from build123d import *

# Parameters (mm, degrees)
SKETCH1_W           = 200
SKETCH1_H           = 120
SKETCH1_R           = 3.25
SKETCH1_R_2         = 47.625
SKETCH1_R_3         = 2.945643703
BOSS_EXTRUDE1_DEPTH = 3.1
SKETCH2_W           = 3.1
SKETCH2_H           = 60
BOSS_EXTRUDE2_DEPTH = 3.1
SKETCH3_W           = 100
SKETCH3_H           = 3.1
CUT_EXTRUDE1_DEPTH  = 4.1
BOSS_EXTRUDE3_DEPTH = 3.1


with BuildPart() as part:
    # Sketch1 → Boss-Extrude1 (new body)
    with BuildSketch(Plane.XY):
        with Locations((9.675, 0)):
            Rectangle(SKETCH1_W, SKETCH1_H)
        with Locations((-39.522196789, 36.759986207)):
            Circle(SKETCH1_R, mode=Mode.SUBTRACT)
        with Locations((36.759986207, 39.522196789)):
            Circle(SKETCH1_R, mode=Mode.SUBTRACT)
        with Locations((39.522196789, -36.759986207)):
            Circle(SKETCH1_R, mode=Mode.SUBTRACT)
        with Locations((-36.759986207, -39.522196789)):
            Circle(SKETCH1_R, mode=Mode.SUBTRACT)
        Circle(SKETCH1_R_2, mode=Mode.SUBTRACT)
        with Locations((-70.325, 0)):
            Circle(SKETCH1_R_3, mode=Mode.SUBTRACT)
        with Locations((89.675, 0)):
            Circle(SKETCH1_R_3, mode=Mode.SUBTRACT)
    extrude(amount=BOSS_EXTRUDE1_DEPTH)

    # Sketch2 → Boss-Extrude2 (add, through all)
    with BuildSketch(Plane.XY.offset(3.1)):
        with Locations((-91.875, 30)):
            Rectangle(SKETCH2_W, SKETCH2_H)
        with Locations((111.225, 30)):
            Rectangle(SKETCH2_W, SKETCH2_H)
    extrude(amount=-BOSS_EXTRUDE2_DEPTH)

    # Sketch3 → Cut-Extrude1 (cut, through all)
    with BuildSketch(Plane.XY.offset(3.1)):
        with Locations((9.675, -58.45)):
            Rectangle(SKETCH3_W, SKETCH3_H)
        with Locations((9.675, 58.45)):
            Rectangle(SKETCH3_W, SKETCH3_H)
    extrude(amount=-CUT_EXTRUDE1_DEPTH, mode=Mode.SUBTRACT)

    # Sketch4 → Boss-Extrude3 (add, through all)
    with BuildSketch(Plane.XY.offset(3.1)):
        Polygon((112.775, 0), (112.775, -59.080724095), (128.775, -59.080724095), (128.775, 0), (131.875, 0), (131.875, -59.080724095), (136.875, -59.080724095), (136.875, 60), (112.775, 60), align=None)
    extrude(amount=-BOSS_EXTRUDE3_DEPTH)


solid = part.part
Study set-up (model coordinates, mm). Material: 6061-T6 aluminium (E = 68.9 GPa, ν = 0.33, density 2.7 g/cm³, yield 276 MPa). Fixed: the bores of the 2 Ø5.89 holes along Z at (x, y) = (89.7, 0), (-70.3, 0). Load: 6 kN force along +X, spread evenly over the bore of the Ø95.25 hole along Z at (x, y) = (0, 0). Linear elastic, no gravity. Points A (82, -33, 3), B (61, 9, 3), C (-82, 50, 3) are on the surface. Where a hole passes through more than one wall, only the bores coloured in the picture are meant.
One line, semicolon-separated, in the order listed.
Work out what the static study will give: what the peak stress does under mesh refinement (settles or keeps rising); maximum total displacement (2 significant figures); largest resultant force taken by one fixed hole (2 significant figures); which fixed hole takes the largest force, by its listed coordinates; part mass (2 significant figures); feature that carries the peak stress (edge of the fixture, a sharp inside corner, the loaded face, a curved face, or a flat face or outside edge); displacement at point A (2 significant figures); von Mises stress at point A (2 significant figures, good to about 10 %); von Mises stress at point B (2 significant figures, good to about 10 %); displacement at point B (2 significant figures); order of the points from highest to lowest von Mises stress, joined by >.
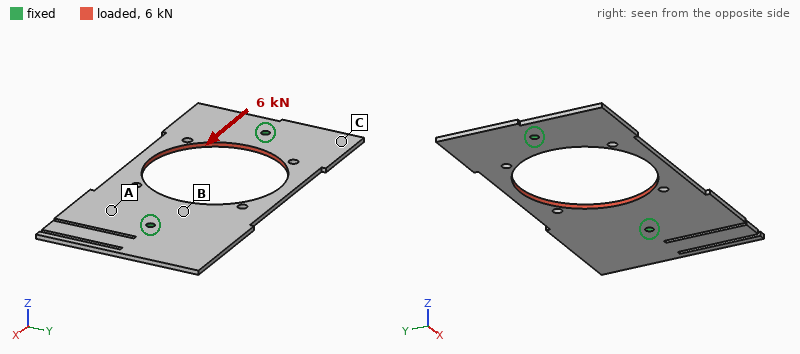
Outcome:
keeps rising; 42 µm; 3.3 kN; (89.7, 0); 160 g; edge of the fixture; 18 µm; 10 MPa; 18 MPa; 12 µm; B > A > C
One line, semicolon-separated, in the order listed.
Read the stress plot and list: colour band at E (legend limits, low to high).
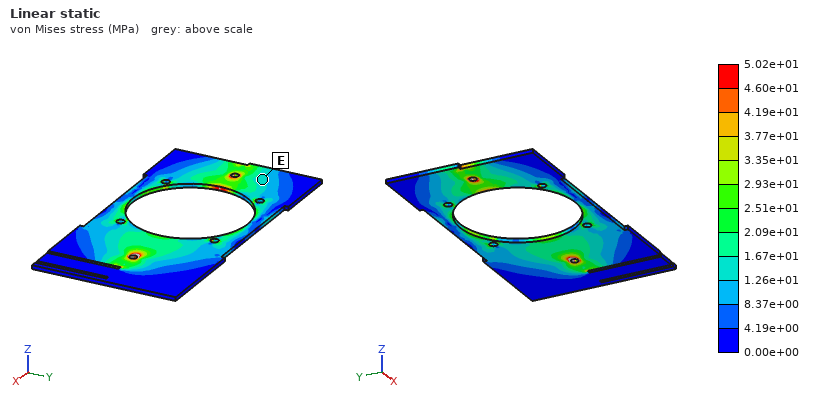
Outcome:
1.26e+01 to 1.67e+01 MPa
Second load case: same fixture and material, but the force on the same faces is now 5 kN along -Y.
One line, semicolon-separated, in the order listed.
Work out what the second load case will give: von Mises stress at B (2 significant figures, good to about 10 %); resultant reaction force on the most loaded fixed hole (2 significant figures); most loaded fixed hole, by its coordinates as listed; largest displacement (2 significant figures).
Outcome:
15 MPa; 2.7 kN; (-70.3, 0); 90 µm
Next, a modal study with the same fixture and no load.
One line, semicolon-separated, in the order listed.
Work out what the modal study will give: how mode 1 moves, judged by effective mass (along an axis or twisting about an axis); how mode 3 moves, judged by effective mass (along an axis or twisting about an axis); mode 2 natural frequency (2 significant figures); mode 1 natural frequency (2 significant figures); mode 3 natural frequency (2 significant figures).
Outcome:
twisting about X; along Z; 460 Hz; 400 Hz; 510 Hz
